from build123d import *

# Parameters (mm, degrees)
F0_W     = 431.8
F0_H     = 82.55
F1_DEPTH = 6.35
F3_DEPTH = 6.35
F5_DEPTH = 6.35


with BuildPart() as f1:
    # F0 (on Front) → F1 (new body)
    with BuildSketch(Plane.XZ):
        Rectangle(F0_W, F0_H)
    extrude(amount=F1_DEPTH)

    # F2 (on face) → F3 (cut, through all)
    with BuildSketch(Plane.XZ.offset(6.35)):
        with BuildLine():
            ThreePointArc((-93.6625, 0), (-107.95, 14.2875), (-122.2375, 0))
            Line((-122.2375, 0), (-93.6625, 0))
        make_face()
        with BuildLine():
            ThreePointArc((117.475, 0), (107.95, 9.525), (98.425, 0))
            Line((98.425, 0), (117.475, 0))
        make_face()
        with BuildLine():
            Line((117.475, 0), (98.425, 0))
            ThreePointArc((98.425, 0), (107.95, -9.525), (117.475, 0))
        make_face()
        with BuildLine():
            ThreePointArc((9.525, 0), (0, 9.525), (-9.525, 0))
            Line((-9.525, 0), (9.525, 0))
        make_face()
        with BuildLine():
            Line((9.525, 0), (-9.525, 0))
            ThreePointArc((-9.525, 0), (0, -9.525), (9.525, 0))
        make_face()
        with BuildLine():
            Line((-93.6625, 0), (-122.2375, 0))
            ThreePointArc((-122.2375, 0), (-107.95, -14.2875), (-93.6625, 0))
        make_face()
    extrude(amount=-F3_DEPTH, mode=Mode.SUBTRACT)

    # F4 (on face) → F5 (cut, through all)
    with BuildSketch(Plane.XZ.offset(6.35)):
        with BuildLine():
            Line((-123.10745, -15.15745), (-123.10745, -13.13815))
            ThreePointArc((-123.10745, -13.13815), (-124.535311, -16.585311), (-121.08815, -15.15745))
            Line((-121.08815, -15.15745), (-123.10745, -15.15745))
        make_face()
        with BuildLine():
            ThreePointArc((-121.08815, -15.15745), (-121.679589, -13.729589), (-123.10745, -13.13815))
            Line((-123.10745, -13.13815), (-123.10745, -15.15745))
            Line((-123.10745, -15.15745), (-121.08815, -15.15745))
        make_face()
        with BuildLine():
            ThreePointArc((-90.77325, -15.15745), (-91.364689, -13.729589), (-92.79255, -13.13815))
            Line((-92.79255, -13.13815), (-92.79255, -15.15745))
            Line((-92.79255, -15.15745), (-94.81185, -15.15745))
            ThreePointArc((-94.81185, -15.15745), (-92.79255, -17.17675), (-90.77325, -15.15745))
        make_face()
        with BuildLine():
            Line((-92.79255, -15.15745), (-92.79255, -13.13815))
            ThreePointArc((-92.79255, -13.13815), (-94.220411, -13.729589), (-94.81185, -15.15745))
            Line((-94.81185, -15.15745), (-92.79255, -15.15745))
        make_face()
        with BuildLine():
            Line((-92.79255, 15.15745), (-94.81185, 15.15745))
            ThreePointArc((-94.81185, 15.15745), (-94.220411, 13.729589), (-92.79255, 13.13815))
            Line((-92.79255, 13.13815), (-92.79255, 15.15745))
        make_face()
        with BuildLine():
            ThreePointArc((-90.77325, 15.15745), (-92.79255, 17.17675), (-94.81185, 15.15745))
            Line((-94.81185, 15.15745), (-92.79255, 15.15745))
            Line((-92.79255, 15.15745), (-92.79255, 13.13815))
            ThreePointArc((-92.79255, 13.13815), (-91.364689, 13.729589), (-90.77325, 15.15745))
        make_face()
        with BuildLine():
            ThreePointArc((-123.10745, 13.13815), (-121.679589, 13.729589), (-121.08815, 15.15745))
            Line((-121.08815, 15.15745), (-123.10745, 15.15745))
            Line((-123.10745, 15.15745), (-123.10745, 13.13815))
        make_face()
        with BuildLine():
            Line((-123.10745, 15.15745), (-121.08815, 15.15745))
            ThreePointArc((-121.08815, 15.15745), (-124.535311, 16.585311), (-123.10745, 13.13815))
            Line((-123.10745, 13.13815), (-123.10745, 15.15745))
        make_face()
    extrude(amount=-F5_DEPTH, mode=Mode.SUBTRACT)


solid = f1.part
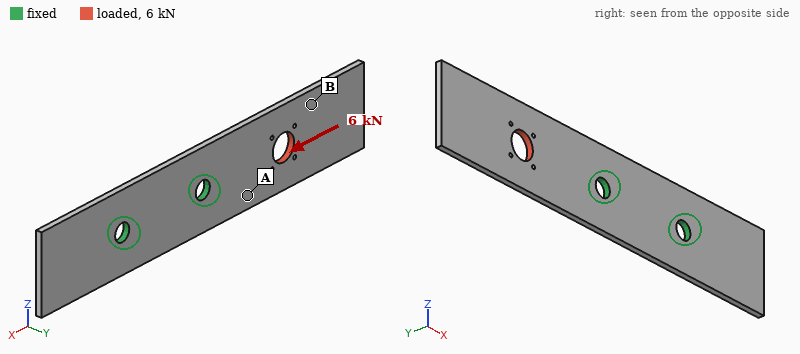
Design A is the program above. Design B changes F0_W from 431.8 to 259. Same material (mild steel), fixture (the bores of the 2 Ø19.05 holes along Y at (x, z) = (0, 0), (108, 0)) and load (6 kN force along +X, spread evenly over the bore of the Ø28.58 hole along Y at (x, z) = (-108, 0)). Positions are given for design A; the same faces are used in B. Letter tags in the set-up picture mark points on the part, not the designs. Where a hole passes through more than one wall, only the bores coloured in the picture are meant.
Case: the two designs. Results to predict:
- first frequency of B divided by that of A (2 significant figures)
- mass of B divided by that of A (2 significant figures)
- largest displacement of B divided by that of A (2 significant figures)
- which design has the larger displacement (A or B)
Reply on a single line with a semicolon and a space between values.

3.2; 0.59; 1.5; B
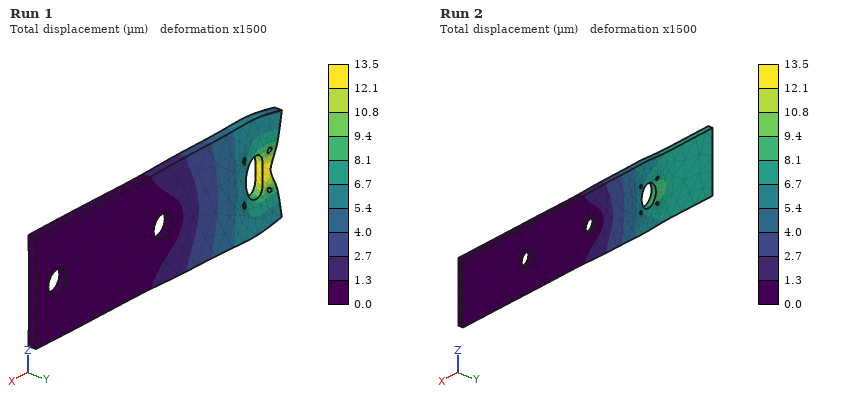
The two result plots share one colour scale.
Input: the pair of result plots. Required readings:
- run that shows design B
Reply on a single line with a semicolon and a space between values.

Run 1
